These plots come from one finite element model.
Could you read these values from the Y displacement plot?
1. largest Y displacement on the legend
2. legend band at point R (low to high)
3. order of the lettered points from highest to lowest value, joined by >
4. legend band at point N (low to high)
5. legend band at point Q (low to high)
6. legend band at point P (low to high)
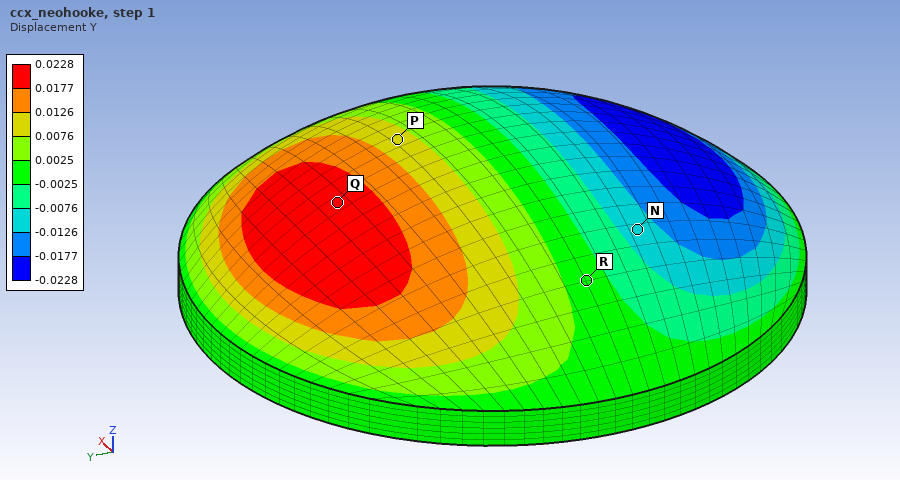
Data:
0.0228
-0.0025 to 0.0025
Q > P > R > N
-0.0126 to -0.0076
0.0177 to 0.0228
0.0076 to 0.0126
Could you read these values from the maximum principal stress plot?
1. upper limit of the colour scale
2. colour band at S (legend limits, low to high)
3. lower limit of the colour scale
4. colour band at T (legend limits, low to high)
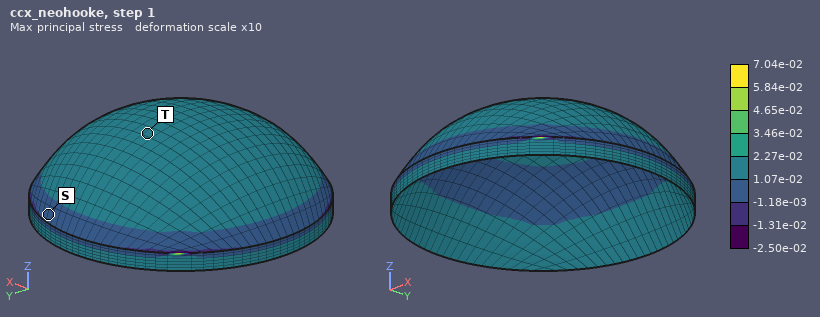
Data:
7.04e-02
-1.18e-03 to 1.07e-02
-2.50e-02
1.07e-02 to 2.27e-02
